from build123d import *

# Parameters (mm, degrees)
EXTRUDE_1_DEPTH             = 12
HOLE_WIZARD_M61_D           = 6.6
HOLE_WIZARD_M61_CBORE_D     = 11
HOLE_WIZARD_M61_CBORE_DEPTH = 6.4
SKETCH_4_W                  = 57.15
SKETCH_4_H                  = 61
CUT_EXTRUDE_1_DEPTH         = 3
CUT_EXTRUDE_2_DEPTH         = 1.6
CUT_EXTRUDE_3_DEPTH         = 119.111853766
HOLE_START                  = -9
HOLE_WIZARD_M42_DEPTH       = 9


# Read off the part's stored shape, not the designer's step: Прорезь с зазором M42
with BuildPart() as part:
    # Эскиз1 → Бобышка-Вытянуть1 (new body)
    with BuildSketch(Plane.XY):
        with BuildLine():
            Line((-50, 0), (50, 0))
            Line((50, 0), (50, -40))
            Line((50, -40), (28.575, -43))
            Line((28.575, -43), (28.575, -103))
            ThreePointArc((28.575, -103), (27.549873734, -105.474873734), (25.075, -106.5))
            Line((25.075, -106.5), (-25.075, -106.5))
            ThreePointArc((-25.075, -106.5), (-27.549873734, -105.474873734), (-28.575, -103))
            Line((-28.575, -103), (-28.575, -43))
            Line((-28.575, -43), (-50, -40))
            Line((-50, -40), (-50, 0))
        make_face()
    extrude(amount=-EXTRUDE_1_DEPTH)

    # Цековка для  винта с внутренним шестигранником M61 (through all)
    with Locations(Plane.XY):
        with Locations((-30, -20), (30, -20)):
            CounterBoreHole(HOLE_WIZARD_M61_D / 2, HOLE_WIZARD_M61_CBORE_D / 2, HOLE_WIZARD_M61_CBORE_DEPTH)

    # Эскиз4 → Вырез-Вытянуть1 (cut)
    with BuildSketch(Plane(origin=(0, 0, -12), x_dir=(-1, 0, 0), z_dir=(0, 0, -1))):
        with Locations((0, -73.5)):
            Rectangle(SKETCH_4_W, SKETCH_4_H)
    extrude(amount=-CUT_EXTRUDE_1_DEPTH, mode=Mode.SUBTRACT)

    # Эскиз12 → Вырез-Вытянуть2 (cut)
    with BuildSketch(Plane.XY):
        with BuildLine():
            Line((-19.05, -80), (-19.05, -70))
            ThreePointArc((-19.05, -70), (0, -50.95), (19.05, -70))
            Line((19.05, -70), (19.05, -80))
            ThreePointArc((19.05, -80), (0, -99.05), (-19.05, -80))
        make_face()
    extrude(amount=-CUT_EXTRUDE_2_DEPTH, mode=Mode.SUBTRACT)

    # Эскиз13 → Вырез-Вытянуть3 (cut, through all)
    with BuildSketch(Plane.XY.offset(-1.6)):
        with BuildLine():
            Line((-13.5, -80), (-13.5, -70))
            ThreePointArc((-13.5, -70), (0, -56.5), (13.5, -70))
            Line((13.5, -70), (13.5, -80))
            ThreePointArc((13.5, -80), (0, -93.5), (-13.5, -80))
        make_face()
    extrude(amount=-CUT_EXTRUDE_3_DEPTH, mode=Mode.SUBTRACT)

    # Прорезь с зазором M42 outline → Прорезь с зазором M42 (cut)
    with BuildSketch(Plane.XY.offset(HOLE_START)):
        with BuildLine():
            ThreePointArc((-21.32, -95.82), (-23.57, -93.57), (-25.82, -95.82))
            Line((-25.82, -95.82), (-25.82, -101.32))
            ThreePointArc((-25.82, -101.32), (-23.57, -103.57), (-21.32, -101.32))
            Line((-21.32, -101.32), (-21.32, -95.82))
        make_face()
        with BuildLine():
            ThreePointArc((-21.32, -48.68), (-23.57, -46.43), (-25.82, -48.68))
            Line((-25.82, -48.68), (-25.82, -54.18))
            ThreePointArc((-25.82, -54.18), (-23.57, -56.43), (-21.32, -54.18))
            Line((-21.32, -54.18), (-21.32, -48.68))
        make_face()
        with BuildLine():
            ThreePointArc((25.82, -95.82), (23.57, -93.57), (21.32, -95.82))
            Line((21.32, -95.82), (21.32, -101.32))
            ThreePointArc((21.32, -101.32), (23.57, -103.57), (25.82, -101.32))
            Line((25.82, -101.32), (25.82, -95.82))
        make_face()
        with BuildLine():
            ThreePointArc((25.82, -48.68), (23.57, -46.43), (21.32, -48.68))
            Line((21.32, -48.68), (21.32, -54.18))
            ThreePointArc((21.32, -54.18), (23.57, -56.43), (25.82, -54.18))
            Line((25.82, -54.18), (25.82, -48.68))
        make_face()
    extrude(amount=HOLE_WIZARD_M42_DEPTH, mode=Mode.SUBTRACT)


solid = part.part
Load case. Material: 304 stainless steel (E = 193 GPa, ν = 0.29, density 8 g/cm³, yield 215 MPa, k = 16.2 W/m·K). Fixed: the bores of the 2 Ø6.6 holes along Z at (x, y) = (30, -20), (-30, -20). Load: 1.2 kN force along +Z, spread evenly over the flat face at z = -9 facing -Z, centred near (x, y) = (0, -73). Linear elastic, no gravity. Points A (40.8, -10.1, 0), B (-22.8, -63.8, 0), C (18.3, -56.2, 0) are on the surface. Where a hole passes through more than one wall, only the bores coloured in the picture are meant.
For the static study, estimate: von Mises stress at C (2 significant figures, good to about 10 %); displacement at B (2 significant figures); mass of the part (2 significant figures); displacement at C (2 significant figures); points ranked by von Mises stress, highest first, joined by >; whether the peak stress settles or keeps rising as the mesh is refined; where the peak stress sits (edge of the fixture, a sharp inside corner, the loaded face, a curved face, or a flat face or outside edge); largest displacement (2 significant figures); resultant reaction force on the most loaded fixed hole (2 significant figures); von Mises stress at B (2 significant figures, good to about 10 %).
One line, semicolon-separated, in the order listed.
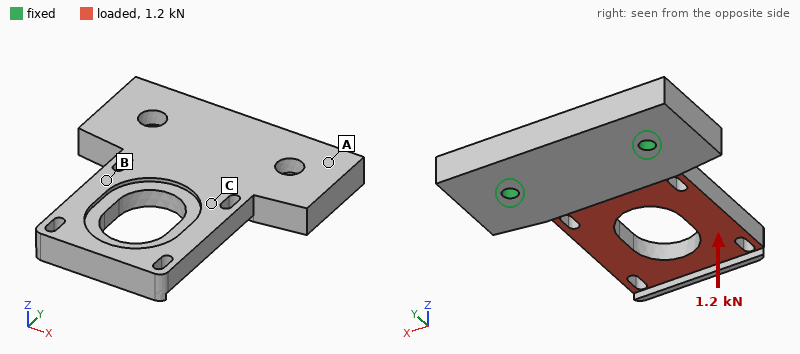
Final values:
56 MPa; 0.074 mm; 580 g; 0.055 mm; C > B > A; keeps rising; edge of the fixture; 0.22 mm; 860 N; 42 MPa
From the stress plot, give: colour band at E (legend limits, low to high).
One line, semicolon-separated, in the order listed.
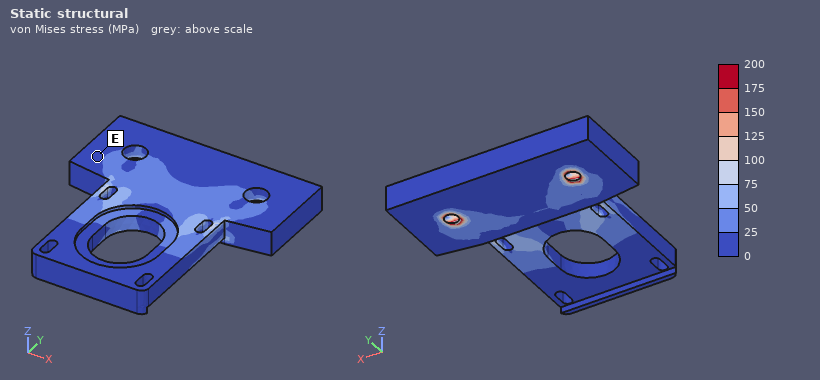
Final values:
0 to 25 MPa
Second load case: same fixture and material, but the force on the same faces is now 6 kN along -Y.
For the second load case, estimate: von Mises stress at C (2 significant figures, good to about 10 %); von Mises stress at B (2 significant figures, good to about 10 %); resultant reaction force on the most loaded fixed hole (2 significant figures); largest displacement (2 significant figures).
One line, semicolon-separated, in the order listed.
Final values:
31 MPa; 31 MPa; 3.1 kN; 0.11 mm
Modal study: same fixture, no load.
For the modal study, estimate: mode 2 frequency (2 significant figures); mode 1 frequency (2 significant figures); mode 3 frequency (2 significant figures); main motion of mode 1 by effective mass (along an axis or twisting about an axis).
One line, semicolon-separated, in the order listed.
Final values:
2900 Hz; 1000 Hz; 4200 Hz; along Z
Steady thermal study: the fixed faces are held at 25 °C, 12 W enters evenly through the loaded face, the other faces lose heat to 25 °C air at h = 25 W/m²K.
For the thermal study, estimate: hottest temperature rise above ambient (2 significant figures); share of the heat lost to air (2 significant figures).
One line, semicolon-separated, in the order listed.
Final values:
43 K; 60 %
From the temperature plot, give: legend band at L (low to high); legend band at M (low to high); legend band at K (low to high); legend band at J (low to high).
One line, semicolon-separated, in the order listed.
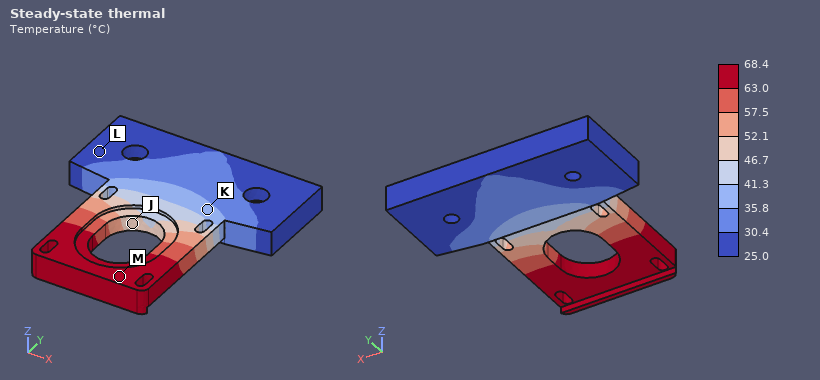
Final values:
25.0 to 30.4 °C; 63.0 to 68.4 °C; 35.8 to 41.3 °C; 46.7 to 52.1 °C
